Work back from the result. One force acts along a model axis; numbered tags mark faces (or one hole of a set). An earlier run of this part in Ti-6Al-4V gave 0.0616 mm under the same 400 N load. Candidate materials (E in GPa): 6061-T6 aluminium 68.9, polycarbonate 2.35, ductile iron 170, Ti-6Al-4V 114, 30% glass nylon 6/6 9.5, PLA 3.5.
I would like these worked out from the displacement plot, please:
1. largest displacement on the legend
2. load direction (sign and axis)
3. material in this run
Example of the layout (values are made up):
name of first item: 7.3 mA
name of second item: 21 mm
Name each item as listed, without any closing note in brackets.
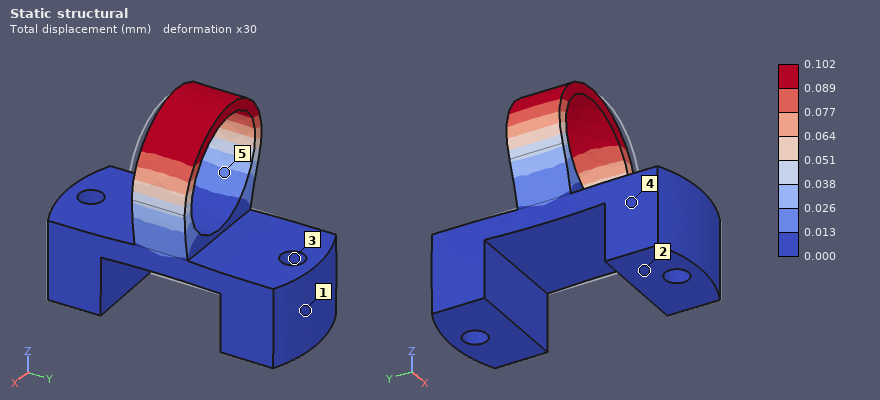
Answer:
largest displacement on the legend: 0.102 mm
load direction: -X
material in this run: 6061-T6 aluminium
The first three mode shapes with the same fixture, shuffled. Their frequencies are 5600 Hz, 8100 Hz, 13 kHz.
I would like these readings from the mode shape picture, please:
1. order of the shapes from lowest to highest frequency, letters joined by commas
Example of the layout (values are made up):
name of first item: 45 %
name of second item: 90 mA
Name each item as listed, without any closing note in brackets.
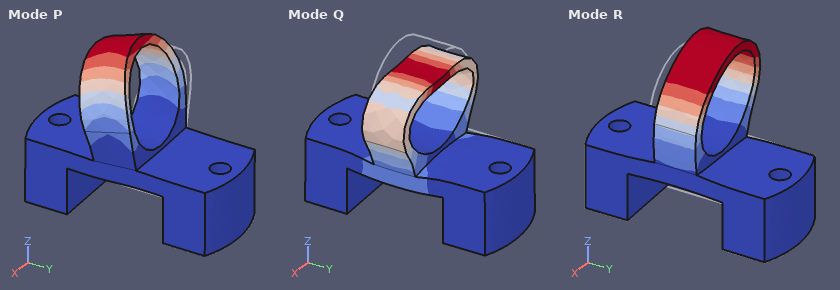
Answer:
order of the shapes from lowest to highest frequency, letters joined by commas: R, P, Q
